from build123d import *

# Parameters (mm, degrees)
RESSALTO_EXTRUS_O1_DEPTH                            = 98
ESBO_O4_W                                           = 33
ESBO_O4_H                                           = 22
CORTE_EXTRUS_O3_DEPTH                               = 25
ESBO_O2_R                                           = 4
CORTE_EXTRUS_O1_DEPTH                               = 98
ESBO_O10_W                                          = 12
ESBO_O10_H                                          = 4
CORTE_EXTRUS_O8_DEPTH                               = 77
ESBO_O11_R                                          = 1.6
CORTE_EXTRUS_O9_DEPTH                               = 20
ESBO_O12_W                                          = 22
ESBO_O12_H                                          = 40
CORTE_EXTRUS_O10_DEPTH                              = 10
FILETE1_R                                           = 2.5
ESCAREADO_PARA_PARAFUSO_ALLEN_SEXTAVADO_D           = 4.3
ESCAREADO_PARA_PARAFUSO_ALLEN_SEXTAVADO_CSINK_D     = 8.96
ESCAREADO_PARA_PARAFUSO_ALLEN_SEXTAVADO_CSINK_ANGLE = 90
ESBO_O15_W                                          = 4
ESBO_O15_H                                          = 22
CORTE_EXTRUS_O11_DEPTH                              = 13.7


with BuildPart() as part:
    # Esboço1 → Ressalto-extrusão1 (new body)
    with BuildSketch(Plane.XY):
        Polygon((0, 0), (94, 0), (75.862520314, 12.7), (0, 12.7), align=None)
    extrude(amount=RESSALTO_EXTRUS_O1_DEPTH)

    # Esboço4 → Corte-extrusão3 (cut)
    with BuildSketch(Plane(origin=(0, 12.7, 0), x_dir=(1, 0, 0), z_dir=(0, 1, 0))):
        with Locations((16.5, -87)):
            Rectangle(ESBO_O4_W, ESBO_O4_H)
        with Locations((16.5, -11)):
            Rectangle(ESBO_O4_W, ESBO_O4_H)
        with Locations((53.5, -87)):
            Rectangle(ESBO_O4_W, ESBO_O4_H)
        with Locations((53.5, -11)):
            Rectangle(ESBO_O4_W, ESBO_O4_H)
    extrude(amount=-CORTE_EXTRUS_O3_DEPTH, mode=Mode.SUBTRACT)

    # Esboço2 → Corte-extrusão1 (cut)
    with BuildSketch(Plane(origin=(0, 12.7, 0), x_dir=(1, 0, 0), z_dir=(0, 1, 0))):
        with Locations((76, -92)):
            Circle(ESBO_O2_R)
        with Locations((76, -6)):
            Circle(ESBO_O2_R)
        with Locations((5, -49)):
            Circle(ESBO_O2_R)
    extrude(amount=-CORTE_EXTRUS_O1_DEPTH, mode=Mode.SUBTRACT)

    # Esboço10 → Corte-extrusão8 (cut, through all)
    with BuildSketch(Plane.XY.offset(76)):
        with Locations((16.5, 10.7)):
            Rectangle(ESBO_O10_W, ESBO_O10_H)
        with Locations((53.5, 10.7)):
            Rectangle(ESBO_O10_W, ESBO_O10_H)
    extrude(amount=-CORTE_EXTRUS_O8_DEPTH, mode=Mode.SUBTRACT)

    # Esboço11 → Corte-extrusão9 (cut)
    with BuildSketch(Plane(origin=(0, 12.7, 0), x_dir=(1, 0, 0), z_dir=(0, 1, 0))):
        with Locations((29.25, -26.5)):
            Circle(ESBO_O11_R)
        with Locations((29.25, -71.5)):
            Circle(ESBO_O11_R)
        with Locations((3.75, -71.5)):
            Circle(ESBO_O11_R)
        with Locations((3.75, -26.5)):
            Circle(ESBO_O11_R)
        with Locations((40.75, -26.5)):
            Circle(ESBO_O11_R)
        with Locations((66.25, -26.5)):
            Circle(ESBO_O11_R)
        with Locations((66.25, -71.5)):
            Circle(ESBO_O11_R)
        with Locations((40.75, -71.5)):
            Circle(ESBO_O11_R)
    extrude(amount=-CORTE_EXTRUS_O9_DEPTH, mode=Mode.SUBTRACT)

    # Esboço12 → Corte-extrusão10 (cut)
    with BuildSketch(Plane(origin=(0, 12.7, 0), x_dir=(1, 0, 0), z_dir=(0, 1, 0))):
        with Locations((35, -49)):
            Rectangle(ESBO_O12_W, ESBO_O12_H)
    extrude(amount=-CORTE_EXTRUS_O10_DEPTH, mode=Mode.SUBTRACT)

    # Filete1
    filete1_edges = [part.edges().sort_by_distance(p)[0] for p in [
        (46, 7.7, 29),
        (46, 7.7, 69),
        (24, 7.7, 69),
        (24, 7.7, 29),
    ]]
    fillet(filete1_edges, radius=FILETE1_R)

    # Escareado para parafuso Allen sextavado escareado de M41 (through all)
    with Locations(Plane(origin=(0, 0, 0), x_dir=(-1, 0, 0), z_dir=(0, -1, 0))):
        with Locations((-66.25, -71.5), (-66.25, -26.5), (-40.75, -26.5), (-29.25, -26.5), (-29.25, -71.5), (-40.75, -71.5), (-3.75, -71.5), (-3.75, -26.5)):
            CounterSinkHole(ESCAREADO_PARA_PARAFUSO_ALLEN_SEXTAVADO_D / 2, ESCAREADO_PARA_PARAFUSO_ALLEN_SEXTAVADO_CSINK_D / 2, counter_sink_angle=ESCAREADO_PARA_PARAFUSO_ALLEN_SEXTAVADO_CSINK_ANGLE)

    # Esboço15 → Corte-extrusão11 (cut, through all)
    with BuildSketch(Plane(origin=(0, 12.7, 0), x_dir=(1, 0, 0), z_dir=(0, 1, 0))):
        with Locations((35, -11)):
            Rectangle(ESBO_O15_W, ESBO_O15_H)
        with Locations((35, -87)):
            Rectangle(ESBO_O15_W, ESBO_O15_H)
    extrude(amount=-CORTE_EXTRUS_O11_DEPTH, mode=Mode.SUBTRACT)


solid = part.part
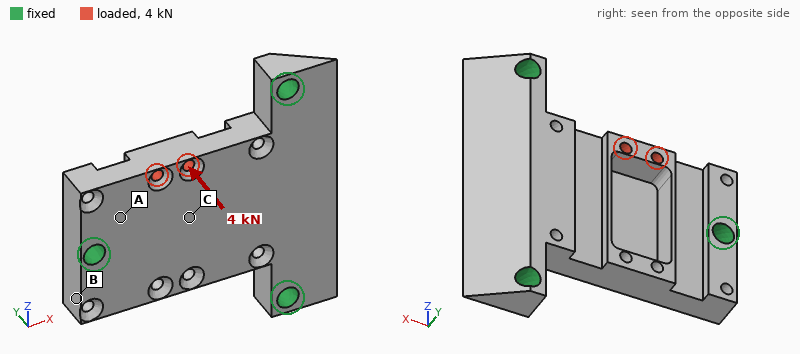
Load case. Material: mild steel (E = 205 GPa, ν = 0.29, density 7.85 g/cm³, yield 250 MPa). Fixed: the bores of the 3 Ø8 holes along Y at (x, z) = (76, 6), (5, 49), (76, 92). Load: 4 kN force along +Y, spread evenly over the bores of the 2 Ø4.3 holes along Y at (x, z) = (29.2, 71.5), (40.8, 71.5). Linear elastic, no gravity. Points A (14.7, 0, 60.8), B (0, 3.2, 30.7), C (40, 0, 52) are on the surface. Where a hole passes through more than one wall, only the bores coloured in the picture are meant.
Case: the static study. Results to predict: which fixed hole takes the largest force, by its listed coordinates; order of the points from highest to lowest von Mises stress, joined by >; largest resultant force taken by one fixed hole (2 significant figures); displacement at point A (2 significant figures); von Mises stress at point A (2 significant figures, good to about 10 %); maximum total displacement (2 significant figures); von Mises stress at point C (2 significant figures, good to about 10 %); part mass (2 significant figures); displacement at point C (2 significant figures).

(5, 49)
A > C > B
2.7 kN
13 µm
74 MPa
57 µm
43 MPa
380 g
26 µm
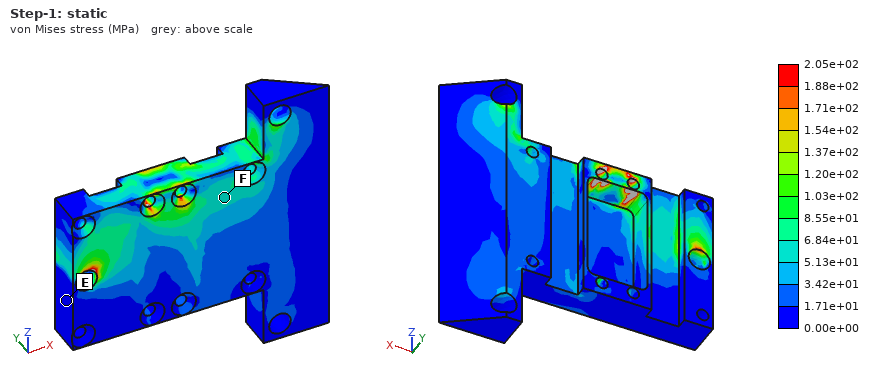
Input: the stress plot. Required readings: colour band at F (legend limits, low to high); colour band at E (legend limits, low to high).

5.13e+01 to 6.84e+01 MPa
0.00e+00 to 1.71e+01 MPa
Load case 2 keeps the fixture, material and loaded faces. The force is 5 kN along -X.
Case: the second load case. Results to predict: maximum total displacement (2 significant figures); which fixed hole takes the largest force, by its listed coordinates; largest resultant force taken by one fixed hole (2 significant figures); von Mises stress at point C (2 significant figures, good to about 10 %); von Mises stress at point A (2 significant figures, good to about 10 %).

13 µm
(5, 49)
3.6 kN
17 MPa
20 MPa
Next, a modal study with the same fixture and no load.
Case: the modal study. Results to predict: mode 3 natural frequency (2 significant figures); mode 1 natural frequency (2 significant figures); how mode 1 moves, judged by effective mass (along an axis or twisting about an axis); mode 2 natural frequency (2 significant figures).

8600 Hz
5300 Hz
along Y
8500 Hz
